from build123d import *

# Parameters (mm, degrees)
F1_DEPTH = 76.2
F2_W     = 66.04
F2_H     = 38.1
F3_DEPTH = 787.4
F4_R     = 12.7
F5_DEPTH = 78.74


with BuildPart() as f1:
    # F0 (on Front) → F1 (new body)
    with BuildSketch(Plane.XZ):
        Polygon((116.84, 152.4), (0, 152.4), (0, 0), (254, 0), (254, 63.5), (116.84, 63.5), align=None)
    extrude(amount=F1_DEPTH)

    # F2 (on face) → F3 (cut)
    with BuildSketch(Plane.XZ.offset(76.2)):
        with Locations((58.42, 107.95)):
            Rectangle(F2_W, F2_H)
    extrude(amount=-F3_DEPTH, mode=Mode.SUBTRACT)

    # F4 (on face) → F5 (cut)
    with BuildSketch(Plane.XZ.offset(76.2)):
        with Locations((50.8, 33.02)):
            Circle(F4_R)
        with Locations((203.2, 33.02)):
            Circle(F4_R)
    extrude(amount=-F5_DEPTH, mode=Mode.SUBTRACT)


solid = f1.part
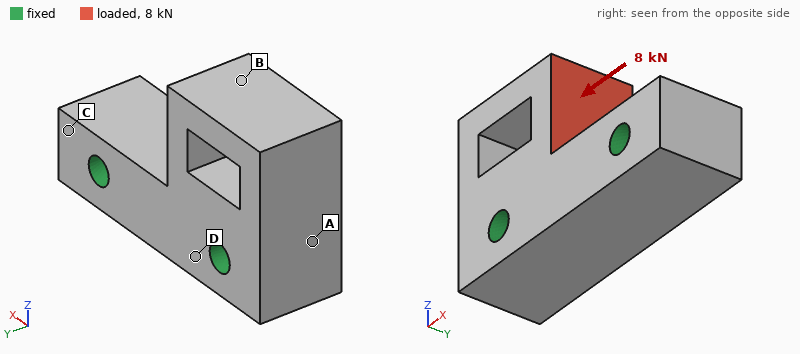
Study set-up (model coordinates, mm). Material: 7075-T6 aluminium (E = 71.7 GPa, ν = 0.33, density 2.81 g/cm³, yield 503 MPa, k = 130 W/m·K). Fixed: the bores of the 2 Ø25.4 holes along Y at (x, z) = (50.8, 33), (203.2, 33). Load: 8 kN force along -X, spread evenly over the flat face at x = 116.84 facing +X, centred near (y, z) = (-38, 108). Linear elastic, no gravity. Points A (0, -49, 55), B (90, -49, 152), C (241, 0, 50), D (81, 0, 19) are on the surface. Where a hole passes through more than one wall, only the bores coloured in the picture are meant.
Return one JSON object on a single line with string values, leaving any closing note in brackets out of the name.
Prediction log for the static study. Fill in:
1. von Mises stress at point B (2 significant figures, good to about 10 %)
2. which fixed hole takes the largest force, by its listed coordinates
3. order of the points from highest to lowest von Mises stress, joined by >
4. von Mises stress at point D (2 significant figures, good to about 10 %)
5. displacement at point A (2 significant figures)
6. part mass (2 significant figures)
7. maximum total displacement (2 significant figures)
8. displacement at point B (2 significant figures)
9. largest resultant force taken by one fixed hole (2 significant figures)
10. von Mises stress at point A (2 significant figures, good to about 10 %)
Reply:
{"von Mises stress at point B": "3.6 MPa", "which fixed hole takes the largest force, by its listed coordinates": "(50.8, 33)", "order of the points from highest to lowest von Mises stress, joined by >": "B > A > D > C", "von Mises stress at point D": "1.5 MPa", "displacement at point A": "4.0 µm", "part mass": "4.9 kg", "maximum total displacement": "20 µm", "displacement at point B": "19 µm", "largest resultant force taken by one fixed hole": "6.8 kN", "von Mises stress at point A": "2.5 MPa"}
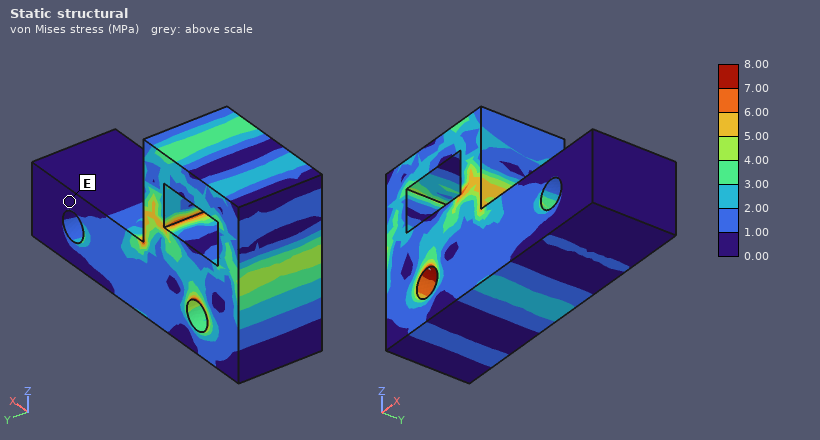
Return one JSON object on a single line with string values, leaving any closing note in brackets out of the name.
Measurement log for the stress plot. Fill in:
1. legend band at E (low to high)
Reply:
{"legend band at E": "0.00 to 1.00 MPa"}
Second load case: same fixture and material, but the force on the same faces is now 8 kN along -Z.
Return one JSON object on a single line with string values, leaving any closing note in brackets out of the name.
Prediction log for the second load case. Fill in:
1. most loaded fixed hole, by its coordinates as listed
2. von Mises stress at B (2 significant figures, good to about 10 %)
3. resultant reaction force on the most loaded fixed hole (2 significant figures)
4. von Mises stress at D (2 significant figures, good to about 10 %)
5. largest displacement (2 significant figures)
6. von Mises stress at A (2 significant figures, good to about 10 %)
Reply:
{"most loaded fixed hole, by its coordinates as listed": "(50.8, 33)", "von Mises stress at B": "2.2 MPa", "resultant reaction force on the most loaded fixed hole": "5.2 kN", "von Mises stress at D": "2.3 MPa", "largest displacement": "15 µm", "von Mises stress at A": "1.3 MPa"}
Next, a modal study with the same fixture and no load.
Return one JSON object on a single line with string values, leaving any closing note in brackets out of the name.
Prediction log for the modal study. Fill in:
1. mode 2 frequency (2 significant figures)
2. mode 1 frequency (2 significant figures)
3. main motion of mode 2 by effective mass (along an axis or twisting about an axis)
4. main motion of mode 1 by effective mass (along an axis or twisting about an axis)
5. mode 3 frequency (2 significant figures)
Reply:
{"mode 2 frequency": "3000 Hz", "mode 1 frequency": "2800 Hz", "main motion of mode 2 by effective mass": "along Y", "main motion of mode 1 by effective mass": "along X", "mode 3 frequency": "4600 Hz"}
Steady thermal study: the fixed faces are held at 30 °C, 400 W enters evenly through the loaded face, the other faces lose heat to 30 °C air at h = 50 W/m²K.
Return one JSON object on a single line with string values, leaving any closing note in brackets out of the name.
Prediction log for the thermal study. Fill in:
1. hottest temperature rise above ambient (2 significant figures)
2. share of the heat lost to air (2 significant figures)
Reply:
{"hottest temperature rise above ambient": "53 K", "share of the heat lost to air": "17 %"}
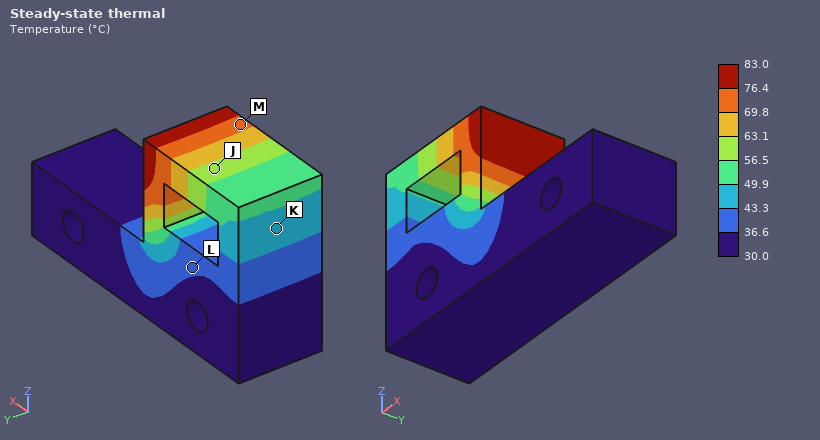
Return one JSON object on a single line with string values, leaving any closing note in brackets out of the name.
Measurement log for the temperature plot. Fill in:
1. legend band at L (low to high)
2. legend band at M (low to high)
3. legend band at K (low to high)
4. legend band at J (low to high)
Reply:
{"legend band at L": "36.6 to 43.3 °C", "legend band at M": "69.8 to 76.4 °C", "legend band at K": "43.3 to 49.9 °C", "legend band at J": "56.5 to 63.1 °C"}
